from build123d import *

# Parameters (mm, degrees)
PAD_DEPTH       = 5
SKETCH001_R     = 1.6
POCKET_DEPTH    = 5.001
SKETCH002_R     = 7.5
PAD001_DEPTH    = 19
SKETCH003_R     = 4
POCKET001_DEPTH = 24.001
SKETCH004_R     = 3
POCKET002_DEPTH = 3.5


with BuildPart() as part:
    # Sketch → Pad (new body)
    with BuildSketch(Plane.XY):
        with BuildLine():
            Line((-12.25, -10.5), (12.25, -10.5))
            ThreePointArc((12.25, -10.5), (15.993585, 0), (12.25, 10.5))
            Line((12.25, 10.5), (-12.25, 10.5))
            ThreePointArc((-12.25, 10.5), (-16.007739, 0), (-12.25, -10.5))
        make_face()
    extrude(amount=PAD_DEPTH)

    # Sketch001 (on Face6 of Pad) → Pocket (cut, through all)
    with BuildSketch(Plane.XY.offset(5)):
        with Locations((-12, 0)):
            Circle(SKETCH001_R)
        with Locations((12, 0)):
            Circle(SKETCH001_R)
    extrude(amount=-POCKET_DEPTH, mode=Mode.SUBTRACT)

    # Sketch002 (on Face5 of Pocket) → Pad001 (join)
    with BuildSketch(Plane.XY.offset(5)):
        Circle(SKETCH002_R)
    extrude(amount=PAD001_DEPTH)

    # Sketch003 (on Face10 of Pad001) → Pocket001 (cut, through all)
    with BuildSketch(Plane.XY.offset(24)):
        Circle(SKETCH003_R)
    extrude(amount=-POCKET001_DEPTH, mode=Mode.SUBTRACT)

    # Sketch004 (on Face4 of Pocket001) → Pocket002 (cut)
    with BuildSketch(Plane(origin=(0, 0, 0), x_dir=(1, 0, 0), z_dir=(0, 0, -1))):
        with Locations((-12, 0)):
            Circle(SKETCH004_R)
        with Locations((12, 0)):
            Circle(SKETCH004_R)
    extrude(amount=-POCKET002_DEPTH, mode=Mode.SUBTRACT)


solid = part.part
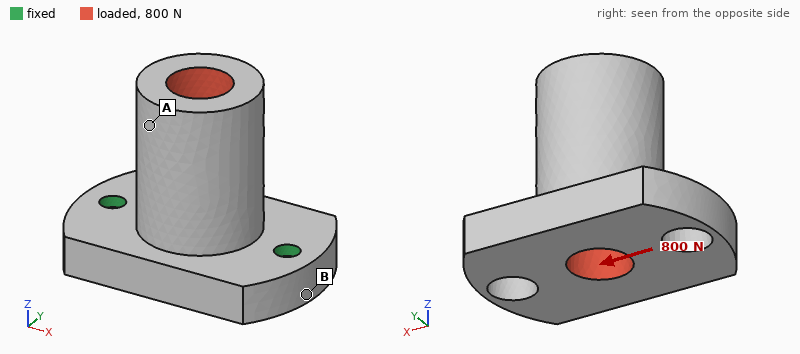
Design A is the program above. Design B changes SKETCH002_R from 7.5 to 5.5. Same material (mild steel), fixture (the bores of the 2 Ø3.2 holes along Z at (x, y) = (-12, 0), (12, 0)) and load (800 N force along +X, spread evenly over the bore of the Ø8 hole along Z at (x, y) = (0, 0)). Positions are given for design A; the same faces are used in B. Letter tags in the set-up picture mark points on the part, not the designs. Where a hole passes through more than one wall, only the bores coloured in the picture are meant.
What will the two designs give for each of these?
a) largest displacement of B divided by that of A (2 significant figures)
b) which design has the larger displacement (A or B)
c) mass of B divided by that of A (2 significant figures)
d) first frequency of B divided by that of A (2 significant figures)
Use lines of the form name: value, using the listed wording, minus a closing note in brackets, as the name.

largest displacement of B divided by that of A: 2.6
which design has the larger displacement: B
mass of B divided by that of A: 0.69
first frequency of B divided by that of A: 1.4
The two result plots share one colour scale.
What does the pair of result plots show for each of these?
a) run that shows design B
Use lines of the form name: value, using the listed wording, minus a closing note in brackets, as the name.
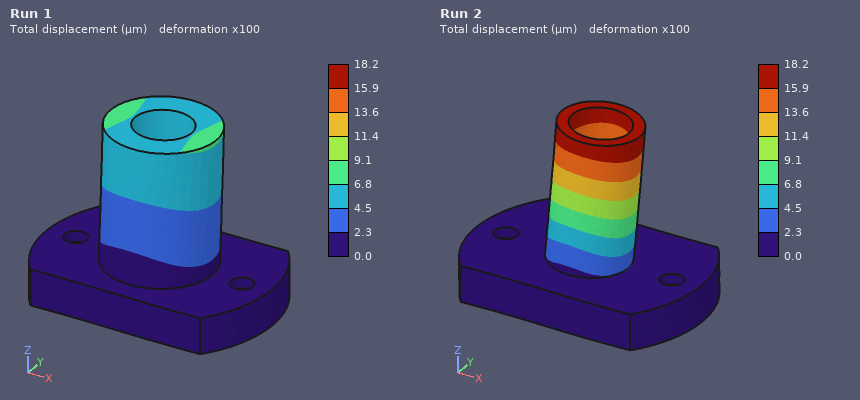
run that shows design B: Run 2
